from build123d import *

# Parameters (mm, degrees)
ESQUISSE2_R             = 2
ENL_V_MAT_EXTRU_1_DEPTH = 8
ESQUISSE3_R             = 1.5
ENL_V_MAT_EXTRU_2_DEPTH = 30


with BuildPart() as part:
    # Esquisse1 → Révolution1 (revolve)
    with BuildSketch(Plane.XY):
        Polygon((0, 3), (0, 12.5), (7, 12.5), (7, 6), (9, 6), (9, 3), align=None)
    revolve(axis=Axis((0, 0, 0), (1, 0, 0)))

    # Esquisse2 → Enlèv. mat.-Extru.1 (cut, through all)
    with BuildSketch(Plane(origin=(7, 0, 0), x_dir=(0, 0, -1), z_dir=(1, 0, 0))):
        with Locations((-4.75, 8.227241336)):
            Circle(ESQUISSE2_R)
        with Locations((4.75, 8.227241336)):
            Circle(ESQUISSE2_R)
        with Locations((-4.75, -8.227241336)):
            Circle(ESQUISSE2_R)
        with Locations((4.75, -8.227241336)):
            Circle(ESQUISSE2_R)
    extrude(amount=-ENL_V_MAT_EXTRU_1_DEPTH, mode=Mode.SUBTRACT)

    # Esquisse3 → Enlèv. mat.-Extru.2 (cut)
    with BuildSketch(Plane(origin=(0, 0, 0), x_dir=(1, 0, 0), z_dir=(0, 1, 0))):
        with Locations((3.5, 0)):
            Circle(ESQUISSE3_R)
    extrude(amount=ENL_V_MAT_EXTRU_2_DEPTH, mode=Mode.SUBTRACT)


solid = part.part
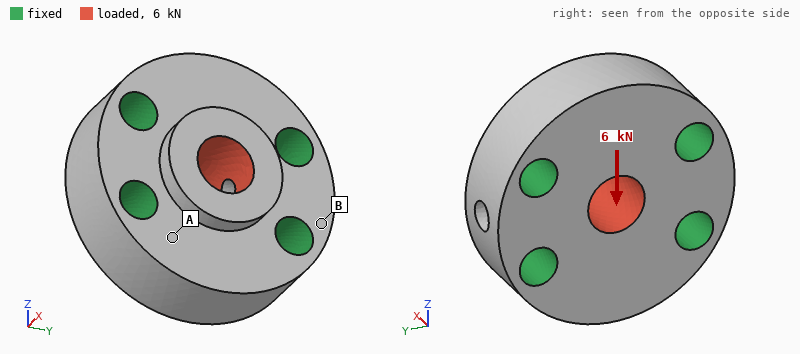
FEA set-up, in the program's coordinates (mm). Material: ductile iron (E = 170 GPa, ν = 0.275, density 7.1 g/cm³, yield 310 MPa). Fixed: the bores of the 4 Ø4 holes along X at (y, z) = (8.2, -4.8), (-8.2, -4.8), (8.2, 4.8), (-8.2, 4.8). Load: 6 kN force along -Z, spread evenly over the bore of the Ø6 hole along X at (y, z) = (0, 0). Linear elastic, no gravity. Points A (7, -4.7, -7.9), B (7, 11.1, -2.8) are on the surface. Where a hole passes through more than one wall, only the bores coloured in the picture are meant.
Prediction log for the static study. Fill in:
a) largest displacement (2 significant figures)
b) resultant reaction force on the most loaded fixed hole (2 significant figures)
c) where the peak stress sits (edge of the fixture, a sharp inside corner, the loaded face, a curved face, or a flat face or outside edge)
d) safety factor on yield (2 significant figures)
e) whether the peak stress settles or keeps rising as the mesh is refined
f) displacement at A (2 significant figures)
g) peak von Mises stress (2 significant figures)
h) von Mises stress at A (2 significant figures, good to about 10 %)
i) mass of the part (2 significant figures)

3.4 µm
1.7 kN
a curved face
2.4
settles
1.0 µm
130 MPa
30 MPa
21 g
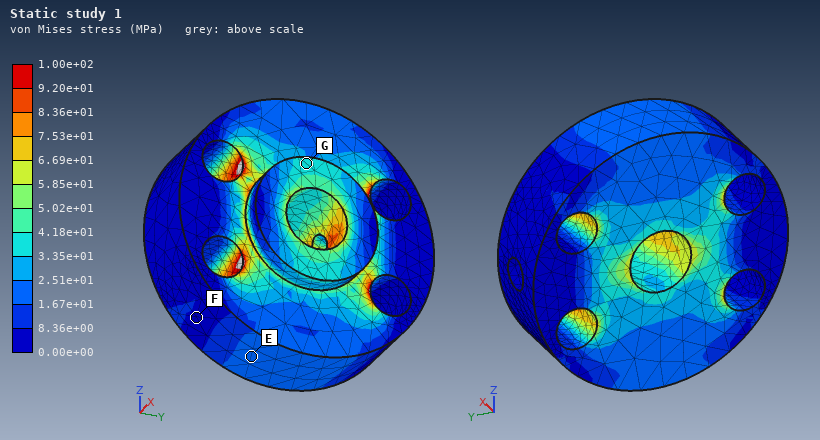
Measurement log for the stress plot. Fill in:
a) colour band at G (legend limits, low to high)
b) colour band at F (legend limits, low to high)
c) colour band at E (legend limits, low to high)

3.35e+01 to 4.18e+01 MPa
0.00e+00 to 8.36e+00 MPa
1.67e+01 to 2.51e+01 MPa
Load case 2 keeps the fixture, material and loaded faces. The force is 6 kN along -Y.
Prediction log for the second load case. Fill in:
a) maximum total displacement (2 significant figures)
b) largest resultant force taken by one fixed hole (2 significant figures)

2.5 µm
1.7 kN
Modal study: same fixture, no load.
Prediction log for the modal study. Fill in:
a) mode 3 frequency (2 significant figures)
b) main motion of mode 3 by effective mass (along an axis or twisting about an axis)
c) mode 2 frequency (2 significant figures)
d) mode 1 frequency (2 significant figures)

93 kHz
along Z
65 kHz
64 kHz
